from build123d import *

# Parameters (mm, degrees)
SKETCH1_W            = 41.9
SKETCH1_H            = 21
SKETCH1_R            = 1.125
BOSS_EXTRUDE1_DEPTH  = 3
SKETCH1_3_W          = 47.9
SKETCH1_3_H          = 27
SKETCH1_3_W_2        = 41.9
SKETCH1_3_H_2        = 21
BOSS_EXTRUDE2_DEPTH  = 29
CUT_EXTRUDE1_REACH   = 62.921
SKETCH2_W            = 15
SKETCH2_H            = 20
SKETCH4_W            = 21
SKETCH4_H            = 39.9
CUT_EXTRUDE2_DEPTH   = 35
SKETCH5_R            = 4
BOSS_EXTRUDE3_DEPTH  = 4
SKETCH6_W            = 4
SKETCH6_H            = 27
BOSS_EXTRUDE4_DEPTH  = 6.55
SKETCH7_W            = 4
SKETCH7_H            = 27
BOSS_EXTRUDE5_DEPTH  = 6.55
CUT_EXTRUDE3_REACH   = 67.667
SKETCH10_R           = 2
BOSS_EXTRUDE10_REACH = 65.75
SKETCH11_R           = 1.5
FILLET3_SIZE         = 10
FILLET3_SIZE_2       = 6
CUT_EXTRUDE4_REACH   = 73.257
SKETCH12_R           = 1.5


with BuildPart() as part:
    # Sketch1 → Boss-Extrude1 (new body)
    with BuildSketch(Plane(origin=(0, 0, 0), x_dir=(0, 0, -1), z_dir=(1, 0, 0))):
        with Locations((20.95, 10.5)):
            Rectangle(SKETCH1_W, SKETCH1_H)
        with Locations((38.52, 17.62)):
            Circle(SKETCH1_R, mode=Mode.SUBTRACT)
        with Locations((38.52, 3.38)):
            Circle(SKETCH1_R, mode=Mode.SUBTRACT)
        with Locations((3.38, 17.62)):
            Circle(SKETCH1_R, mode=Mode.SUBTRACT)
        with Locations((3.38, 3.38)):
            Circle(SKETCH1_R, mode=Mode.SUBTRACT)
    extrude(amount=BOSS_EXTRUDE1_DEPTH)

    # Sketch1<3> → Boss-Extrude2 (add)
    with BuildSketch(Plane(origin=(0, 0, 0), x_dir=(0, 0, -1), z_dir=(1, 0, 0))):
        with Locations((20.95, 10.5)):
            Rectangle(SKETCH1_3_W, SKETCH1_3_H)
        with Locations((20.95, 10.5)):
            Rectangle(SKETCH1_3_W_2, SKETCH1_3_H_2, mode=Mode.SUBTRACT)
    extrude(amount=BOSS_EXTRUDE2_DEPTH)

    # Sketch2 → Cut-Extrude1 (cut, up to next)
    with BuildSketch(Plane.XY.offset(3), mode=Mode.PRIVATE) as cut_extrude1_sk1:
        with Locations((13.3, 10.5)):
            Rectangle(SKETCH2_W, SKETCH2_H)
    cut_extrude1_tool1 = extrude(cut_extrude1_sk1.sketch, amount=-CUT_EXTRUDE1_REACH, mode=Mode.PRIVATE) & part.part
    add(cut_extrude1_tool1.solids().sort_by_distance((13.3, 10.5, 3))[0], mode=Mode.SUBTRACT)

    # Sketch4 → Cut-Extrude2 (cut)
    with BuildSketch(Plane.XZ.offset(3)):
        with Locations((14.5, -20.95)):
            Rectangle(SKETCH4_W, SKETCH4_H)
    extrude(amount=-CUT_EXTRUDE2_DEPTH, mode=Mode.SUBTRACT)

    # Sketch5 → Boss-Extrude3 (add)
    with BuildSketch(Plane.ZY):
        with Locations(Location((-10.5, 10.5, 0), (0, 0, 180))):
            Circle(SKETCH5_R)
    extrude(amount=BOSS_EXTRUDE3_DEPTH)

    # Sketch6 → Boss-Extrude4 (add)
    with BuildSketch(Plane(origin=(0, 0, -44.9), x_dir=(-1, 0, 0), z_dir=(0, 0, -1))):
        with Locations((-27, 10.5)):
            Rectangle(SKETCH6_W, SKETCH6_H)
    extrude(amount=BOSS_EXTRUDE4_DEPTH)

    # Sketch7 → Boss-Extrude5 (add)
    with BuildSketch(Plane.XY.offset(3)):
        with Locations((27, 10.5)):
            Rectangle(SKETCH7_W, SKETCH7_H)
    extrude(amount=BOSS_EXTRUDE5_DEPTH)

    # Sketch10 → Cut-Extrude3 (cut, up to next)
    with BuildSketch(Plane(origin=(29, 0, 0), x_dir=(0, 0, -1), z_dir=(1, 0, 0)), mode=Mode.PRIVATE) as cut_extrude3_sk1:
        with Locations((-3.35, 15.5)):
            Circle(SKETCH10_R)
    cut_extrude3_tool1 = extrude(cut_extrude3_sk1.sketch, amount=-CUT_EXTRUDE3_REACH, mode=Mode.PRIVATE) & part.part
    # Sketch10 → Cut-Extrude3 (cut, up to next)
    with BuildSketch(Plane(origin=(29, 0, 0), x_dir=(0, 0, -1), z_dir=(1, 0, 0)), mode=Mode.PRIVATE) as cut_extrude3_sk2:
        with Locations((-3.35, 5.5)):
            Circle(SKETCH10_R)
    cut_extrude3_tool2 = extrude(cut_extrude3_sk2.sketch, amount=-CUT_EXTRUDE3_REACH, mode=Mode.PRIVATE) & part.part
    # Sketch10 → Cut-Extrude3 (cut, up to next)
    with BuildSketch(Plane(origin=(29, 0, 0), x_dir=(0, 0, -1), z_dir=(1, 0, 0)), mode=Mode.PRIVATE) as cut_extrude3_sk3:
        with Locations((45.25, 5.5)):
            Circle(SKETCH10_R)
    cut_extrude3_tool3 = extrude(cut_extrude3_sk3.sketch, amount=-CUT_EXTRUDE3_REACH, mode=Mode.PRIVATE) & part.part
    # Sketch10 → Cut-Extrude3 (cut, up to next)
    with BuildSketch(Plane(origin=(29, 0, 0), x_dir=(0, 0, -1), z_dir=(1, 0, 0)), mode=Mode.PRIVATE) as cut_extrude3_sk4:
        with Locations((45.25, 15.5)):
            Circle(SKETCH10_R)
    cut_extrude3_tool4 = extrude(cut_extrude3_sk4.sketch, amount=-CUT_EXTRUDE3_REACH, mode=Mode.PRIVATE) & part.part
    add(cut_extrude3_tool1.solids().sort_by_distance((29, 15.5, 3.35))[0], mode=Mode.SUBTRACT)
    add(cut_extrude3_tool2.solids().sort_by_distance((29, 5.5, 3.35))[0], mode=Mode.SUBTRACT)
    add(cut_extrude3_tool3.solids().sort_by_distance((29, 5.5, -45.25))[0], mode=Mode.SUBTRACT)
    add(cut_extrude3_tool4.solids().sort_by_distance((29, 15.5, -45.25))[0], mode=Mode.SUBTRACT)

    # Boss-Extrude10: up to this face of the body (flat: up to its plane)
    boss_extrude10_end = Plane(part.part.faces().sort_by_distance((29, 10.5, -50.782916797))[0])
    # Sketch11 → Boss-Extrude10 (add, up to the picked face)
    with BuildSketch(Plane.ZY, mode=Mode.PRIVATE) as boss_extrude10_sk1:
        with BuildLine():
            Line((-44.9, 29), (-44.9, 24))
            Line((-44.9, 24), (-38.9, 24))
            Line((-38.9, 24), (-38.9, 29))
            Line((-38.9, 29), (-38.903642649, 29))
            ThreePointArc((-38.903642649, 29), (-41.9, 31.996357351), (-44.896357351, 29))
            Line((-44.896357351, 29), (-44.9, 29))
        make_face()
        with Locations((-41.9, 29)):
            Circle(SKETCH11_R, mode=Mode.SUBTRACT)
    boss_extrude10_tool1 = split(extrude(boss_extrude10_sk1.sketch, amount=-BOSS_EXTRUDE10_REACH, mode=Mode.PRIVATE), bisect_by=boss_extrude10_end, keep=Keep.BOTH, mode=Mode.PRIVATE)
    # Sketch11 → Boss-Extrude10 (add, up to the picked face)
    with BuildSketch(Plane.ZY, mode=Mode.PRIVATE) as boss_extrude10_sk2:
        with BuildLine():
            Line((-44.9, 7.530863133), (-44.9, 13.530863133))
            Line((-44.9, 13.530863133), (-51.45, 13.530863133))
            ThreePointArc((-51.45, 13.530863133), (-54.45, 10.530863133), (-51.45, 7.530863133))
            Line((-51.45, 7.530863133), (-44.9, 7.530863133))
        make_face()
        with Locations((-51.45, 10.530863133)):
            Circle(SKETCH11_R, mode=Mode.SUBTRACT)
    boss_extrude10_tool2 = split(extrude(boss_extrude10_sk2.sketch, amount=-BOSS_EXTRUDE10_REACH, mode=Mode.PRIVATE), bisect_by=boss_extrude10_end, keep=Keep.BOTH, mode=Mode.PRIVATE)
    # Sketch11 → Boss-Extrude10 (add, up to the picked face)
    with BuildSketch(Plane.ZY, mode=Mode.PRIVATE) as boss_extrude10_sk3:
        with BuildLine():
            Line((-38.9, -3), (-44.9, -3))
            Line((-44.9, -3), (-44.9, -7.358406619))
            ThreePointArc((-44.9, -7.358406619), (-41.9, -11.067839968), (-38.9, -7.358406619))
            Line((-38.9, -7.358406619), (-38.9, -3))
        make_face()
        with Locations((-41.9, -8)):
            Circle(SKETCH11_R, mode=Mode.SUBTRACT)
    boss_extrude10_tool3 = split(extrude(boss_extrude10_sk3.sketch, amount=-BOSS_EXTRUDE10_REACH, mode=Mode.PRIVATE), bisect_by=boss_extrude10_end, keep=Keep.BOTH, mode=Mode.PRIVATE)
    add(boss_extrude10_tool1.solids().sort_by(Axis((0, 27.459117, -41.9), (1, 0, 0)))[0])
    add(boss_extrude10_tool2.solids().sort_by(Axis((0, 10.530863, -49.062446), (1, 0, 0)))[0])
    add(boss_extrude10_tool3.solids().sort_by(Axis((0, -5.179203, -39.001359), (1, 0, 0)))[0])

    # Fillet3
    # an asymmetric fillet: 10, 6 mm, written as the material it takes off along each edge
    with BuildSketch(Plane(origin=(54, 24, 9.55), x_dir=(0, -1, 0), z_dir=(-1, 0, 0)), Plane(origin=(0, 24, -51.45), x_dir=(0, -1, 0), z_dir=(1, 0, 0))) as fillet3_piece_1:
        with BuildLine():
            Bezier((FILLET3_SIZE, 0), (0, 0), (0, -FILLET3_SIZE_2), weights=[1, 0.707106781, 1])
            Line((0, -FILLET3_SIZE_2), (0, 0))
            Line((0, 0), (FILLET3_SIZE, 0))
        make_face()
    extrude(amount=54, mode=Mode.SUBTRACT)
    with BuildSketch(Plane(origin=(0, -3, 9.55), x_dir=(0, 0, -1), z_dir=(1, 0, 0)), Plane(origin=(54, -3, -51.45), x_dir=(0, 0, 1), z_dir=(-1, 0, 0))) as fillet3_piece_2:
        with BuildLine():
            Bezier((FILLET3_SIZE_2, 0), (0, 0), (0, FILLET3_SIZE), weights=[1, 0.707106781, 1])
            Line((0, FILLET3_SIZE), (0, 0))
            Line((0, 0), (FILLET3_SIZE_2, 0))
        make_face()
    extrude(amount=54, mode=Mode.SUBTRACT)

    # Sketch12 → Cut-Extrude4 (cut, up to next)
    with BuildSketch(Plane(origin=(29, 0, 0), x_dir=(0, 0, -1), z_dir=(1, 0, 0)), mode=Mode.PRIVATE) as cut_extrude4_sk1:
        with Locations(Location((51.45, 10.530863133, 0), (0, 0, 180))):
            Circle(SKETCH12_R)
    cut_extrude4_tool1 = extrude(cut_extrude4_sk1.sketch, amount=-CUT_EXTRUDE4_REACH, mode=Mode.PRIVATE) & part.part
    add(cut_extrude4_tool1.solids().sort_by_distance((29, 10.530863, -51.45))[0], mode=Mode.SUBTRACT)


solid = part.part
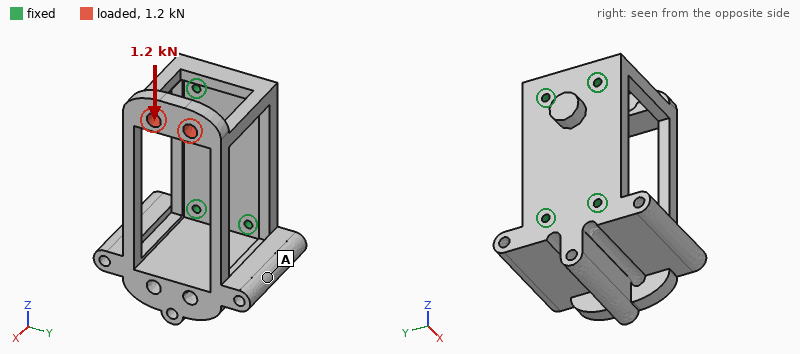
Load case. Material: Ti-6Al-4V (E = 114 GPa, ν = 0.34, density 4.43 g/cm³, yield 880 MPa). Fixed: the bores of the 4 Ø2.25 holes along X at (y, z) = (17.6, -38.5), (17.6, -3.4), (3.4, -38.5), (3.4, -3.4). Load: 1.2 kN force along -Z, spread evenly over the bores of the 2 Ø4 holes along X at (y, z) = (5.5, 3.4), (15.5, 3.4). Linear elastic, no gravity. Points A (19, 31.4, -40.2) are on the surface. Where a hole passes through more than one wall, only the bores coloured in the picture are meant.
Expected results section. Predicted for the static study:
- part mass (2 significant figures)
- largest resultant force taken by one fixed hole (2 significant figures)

57 g
360 N
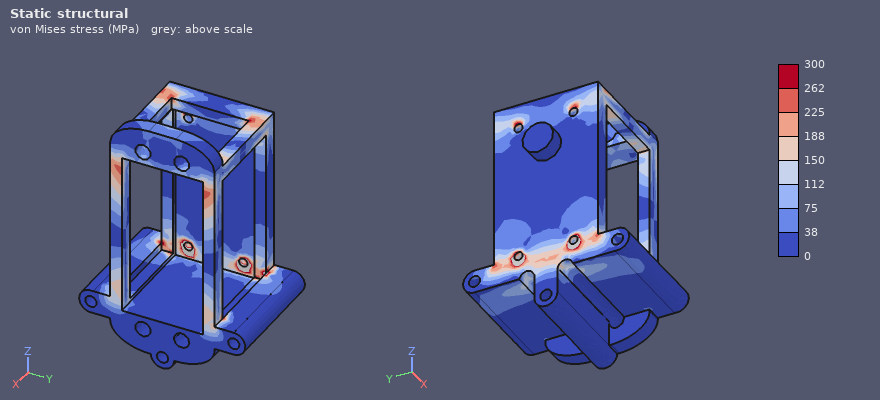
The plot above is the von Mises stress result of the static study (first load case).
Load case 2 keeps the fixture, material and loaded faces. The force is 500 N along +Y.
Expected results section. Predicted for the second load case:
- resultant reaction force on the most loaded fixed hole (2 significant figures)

640 N
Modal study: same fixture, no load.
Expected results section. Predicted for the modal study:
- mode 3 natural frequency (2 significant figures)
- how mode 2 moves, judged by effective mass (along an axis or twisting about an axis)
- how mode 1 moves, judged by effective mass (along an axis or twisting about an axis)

5000 Hz
along Y
along Z
